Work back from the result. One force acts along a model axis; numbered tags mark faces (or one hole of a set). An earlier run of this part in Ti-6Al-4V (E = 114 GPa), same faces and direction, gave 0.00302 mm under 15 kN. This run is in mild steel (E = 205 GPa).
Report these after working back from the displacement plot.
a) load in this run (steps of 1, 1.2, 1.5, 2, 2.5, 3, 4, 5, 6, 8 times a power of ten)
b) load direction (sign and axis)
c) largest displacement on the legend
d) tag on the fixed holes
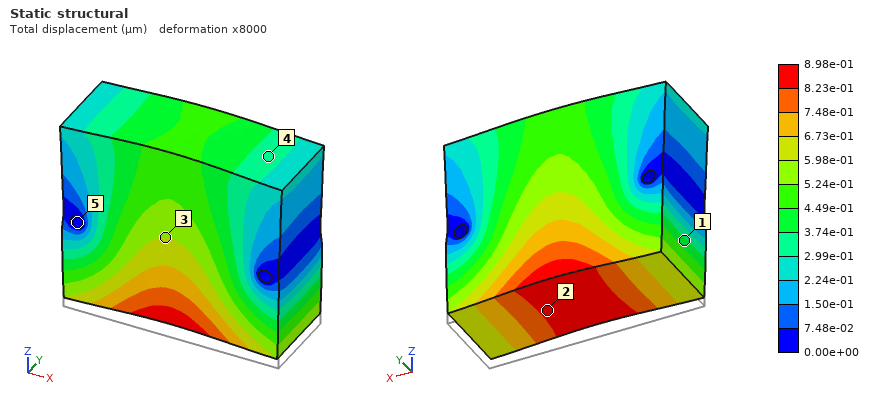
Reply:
8 kN
+Z
8.98e-01 µm
5
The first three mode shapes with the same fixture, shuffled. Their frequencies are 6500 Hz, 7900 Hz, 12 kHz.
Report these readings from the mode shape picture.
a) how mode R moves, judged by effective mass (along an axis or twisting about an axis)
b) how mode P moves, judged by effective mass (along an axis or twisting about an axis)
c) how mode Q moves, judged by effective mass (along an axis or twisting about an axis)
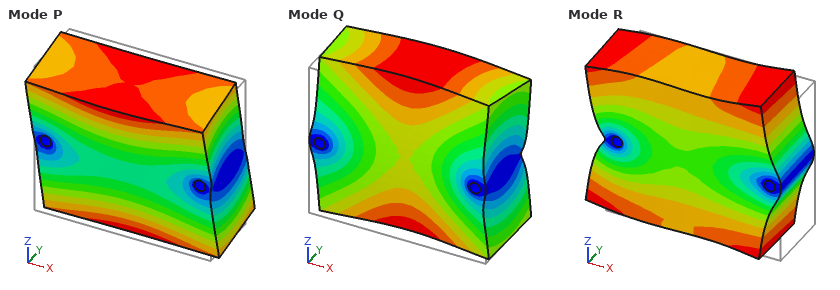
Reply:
along X
twisting about X
along Y
